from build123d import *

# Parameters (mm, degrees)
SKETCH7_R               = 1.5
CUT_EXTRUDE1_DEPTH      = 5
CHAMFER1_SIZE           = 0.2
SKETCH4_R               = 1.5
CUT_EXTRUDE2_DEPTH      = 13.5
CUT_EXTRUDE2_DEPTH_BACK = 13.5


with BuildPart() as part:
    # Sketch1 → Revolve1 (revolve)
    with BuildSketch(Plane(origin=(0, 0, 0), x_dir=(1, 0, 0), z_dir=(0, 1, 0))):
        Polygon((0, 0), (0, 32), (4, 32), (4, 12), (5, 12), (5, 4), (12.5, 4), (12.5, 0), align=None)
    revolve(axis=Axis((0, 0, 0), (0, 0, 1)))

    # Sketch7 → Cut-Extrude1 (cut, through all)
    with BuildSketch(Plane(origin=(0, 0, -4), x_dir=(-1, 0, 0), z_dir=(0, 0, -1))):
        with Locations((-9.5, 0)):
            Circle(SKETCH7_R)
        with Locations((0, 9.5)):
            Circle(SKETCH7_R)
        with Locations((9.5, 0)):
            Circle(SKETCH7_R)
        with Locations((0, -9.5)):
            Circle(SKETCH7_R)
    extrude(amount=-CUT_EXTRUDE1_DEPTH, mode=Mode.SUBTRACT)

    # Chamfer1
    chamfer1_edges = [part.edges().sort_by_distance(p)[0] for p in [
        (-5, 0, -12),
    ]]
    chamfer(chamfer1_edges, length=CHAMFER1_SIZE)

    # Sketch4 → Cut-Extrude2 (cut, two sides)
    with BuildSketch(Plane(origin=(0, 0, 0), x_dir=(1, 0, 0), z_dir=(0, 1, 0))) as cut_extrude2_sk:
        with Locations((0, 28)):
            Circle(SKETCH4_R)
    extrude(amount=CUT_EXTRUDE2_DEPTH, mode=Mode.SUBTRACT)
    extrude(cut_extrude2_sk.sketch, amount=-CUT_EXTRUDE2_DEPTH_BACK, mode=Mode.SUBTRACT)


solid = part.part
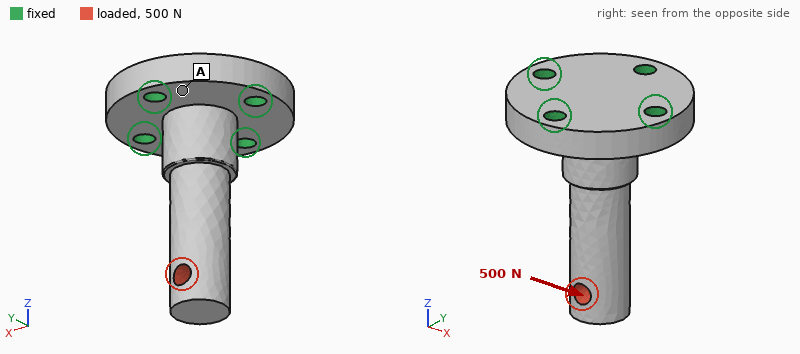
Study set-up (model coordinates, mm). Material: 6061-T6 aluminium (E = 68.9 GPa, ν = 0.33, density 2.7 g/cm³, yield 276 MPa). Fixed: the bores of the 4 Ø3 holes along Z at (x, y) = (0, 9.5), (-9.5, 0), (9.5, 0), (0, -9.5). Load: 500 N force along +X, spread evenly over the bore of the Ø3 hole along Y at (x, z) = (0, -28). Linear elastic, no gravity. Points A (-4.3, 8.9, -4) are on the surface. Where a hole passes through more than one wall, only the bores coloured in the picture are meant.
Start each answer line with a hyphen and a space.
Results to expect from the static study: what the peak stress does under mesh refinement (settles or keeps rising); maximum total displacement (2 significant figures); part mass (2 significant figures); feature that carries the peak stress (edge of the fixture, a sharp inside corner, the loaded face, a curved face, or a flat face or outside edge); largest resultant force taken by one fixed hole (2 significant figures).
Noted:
- keeps rising
- 0.18 mm
- 9.3 g
- a sharp inside corner
- 790 N
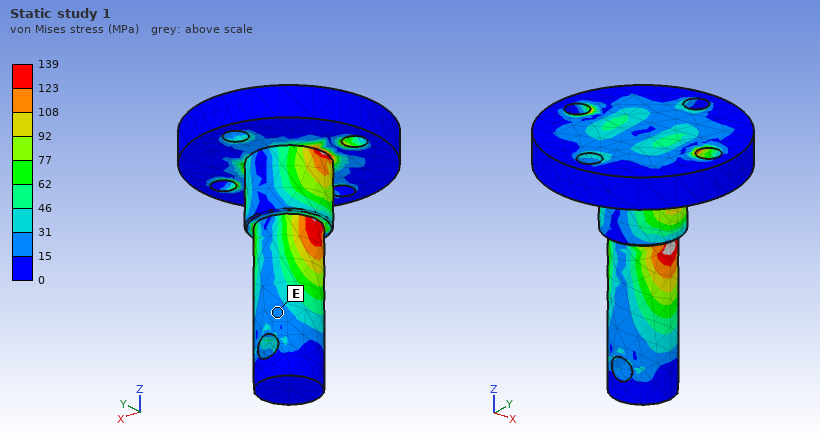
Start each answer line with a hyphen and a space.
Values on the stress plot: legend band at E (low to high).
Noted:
- 15 to 31 MPa
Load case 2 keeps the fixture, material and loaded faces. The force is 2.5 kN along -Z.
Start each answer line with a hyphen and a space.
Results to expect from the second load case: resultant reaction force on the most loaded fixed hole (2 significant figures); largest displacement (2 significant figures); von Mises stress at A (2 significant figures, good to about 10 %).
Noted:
- 650 N
- 26 µm
- 12 MPa
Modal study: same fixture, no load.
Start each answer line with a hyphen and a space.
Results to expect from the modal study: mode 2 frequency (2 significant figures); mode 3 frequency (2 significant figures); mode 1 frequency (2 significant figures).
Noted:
- 8000 Hz
- 32 kHz
- 8000 Hz
